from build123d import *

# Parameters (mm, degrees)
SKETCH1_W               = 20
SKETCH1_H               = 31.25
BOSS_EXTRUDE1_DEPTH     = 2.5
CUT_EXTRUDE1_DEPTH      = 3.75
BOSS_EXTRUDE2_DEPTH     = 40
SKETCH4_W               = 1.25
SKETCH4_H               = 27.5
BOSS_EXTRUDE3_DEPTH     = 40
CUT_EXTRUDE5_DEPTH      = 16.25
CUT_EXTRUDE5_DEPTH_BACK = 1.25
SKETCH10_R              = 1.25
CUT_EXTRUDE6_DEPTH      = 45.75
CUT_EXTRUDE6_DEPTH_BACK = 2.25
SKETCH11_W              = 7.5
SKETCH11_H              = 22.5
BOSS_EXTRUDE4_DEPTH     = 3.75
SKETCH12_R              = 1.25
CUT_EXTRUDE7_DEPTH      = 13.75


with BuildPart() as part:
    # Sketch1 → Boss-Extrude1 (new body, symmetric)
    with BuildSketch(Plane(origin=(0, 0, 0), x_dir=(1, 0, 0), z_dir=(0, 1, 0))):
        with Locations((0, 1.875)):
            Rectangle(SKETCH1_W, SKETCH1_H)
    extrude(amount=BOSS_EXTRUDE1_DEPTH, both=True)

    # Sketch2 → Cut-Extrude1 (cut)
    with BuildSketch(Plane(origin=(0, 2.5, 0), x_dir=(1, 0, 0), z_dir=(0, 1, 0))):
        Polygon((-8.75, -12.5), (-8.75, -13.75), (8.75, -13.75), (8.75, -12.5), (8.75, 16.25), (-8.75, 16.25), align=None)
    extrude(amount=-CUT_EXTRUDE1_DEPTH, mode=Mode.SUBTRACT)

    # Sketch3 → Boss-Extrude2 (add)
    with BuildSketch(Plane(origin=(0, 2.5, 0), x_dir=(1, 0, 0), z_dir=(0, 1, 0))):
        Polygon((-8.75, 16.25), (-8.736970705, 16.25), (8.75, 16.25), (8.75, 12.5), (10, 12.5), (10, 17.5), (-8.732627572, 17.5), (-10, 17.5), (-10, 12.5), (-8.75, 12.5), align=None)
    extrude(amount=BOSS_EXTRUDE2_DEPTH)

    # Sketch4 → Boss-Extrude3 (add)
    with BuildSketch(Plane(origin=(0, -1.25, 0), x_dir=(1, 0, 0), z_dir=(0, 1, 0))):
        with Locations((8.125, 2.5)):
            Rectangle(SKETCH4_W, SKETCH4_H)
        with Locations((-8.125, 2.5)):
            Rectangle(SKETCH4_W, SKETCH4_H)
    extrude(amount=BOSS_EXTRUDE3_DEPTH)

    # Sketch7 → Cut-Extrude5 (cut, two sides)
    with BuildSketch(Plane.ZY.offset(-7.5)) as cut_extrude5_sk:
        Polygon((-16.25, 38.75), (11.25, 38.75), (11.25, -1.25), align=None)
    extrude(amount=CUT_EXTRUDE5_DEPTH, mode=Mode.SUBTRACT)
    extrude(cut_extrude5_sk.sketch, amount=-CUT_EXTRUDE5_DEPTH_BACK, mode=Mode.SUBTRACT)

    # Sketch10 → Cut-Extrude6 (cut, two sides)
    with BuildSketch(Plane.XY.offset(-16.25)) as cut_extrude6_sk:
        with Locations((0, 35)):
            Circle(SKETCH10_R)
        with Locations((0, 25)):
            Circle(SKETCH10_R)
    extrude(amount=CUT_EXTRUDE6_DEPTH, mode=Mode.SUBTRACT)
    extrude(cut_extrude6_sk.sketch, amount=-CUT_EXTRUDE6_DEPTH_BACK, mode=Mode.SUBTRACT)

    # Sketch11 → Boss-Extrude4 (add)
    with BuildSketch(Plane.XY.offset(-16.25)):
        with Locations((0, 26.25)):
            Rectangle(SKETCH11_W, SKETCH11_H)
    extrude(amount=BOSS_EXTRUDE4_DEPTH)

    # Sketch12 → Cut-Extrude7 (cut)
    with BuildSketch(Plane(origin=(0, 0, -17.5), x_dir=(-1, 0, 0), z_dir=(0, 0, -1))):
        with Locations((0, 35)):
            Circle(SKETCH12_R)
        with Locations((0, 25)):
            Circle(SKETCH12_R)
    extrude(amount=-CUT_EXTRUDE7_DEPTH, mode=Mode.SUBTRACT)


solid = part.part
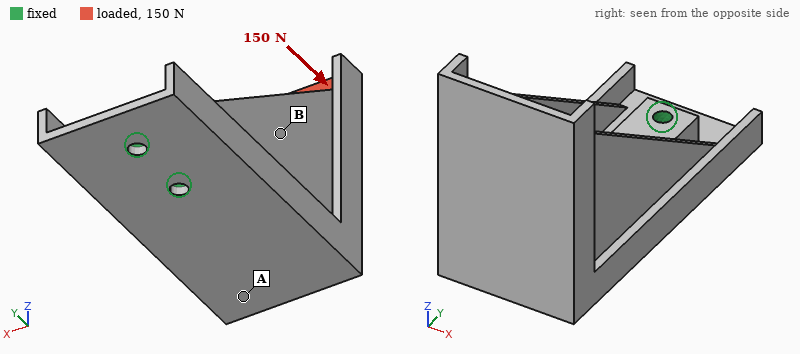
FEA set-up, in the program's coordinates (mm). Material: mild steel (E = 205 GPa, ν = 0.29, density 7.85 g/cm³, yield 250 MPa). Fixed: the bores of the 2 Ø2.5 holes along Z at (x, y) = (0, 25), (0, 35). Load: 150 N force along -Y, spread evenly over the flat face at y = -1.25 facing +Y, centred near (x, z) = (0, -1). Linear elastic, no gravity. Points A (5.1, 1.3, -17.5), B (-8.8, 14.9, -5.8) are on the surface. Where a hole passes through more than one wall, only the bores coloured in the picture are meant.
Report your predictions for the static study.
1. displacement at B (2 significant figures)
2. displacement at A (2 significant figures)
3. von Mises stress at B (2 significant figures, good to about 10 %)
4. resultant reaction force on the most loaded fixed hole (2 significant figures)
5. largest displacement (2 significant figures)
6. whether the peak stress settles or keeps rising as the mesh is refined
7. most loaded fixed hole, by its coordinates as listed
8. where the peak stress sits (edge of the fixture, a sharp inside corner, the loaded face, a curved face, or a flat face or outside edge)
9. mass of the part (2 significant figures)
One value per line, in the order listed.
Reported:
8.3 µm
14 µm
10 MPa
180 N
31 µm
keeps rising
(0, 25)
edge of the fixture
35 g
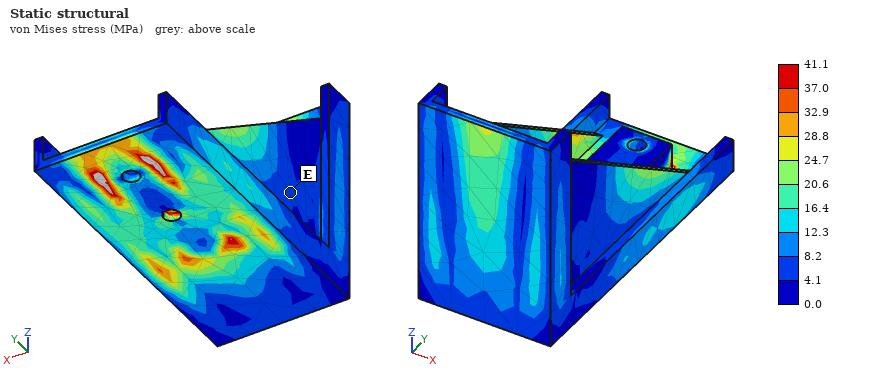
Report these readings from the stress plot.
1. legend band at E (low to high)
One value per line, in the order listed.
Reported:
4.1 to 8.2 MPa
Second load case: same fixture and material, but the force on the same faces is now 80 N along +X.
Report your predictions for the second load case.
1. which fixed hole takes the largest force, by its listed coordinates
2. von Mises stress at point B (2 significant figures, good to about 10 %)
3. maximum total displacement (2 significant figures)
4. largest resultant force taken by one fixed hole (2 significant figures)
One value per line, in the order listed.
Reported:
(0, 25)
16 MPa
100 µm
230 N
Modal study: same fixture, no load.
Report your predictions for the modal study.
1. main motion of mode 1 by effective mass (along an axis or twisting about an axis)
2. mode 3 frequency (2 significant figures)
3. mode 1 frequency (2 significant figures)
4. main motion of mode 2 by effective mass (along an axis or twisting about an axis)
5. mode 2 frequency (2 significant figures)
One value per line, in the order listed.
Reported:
along X
6200 Hz
1500 Hz
along Z
2500 Hz
